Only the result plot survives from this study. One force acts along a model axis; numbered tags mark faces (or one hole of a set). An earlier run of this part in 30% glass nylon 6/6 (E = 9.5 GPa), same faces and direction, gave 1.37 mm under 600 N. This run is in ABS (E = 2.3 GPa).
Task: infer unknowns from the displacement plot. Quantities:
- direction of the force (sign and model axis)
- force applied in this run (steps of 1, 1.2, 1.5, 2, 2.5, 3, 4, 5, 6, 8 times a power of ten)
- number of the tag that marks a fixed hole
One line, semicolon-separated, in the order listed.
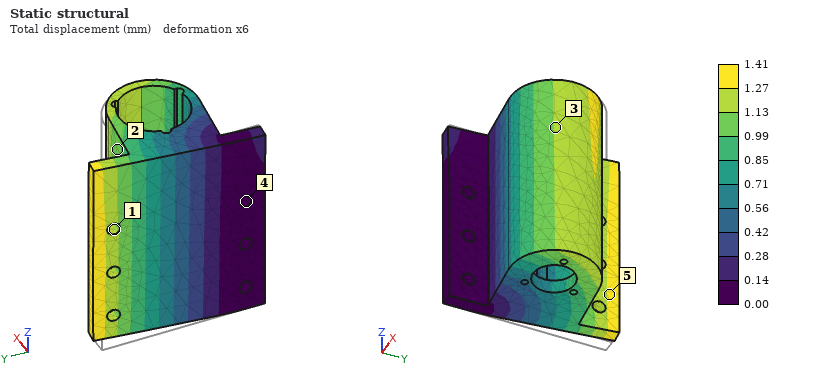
+X; 150 N; 4
